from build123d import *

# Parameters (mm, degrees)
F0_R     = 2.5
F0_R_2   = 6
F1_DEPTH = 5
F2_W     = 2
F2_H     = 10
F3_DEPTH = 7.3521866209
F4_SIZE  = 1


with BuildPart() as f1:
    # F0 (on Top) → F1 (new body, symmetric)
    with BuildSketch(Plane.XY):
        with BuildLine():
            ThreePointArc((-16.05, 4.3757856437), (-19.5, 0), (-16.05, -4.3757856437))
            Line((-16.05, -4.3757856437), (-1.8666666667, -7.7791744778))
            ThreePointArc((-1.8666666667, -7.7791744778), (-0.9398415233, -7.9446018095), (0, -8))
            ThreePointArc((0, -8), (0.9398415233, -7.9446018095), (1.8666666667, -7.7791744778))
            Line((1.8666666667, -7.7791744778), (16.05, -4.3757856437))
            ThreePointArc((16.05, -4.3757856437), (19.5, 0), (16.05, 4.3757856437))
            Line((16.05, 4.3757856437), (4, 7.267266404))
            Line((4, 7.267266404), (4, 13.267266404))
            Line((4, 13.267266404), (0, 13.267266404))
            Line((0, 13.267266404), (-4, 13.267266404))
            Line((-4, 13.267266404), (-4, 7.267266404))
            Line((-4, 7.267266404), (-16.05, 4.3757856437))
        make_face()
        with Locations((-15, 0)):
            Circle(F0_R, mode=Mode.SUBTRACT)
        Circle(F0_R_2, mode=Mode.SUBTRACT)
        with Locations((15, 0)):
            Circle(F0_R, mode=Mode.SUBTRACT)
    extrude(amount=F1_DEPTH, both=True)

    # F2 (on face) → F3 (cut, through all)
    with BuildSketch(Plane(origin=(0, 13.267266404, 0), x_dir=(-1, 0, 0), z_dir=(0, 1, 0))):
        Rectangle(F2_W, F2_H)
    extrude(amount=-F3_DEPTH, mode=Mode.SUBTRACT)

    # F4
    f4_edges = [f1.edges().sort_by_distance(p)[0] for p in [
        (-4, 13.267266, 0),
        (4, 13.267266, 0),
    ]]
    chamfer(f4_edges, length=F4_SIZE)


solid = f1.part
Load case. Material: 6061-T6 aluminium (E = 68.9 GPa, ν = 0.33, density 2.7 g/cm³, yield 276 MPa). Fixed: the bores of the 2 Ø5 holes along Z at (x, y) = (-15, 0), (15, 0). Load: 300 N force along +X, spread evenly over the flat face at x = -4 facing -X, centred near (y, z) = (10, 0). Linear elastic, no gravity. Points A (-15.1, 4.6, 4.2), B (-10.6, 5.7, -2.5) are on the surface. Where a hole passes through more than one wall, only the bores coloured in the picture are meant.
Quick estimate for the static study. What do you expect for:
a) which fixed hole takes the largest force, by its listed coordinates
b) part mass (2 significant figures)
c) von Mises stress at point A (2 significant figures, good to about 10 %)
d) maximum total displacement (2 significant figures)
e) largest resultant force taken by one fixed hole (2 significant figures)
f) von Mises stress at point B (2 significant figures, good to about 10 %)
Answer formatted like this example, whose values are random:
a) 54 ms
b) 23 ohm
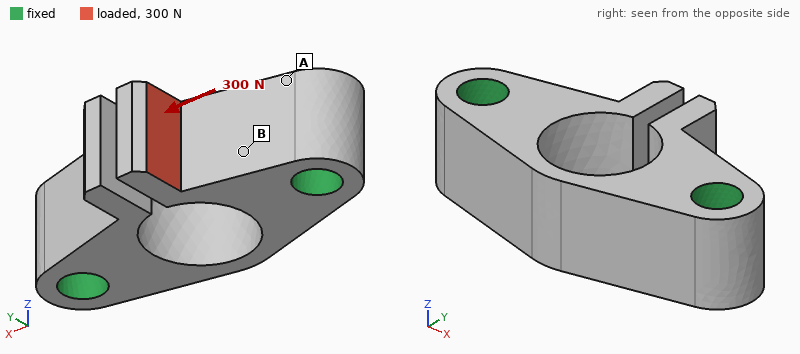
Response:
a) (-15, 0)
b) 8.8 g
c) 11 MPa
d) 51 µm
e) 340 N
f) 29 MPa
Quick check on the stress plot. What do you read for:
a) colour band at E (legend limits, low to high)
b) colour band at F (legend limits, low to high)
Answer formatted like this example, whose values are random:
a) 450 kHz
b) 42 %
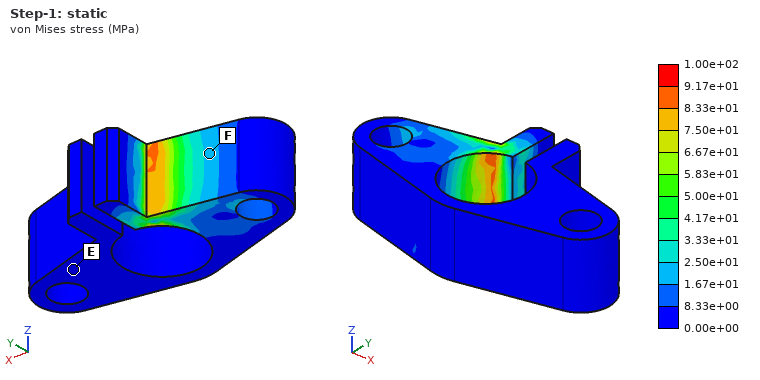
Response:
a) 0.00e+00 to 8.33e+00 MPa
b) 1.67e+01 to 2.50e+01 MPa
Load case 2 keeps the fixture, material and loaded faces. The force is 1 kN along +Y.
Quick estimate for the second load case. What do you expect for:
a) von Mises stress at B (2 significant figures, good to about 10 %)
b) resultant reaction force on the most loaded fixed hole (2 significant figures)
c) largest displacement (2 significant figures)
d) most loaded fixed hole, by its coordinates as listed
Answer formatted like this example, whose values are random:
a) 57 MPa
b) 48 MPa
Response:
a) 54 MPa
b) 960 N
c) 37 µm
d) (-15, 0)
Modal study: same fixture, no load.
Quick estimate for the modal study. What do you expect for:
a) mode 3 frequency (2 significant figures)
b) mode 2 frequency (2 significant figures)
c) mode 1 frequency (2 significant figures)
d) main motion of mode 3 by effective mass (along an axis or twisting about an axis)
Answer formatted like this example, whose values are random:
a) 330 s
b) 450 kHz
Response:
a) 26 kHz
b) 18 kHz
c) 18 kHz
d) along Z
